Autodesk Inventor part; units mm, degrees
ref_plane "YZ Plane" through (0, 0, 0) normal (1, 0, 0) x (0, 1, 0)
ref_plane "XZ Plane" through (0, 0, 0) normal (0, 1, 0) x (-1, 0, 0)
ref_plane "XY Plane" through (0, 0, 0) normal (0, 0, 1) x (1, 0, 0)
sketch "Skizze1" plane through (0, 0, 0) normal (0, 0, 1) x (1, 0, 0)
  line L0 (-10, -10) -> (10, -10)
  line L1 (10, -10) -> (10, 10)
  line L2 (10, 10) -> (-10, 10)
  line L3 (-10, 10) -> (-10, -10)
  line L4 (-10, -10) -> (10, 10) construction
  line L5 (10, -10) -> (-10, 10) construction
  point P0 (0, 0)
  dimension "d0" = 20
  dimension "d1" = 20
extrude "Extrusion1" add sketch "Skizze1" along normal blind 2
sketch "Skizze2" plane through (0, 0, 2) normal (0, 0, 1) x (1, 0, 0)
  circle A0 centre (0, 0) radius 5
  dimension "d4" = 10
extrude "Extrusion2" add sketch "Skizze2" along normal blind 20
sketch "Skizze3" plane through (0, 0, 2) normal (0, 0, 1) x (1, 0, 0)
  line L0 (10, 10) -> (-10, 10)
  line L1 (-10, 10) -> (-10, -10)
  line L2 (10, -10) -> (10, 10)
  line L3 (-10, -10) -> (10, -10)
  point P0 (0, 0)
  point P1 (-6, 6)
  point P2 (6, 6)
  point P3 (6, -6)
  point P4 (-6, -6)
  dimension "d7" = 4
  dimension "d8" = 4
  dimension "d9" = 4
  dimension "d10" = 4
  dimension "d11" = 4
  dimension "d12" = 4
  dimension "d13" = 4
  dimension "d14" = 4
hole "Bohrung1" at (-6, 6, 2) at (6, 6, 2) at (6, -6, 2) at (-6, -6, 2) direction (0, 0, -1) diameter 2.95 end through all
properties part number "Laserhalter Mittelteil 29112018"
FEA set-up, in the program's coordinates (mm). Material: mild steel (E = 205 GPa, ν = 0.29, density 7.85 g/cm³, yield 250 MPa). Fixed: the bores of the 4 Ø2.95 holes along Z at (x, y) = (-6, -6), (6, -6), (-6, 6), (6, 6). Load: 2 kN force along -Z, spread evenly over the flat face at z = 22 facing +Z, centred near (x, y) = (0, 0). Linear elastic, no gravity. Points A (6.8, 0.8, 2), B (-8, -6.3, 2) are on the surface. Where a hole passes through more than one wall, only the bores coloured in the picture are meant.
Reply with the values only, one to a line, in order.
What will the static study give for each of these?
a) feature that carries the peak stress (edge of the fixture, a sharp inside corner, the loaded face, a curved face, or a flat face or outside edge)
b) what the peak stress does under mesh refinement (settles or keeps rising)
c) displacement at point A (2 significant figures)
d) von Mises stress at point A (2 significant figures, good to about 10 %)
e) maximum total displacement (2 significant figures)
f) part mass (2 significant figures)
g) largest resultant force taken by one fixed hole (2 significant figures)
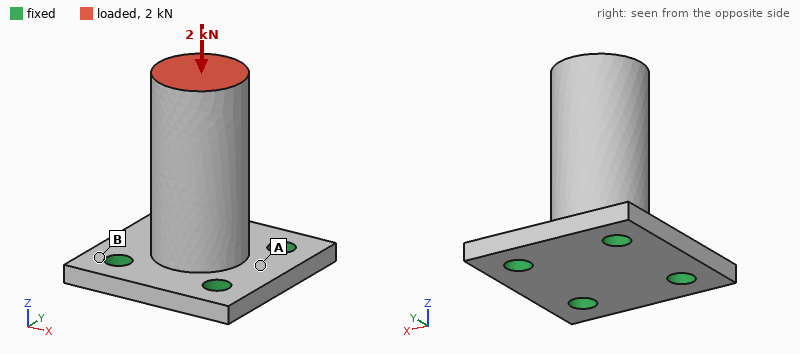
edge of the fixture
keeps rising
2.1 µm
40 MPa
6.4 µm
18 g
530 N
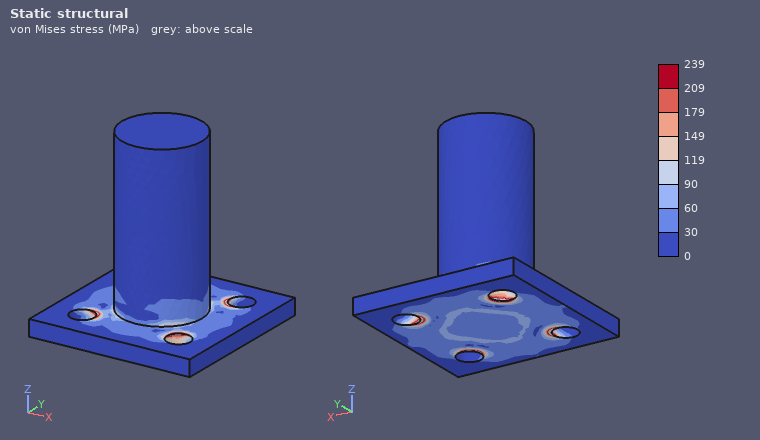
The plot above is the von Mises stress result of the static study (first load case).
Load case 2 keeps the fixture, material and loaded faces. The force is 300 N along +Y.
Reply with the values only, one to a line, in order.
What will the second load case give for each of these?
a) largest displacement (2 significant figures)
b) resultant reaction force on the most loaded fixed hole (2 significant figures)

22 µm
330 N
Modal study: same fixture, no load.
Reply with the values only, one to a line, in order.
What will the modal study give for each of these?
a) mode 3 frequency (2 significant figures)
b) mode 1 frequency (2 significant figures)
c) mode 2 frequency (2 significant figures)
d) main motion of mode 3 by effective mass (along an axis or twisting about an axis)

28 kHz
9600 Hz
9600 Hz
along Z
